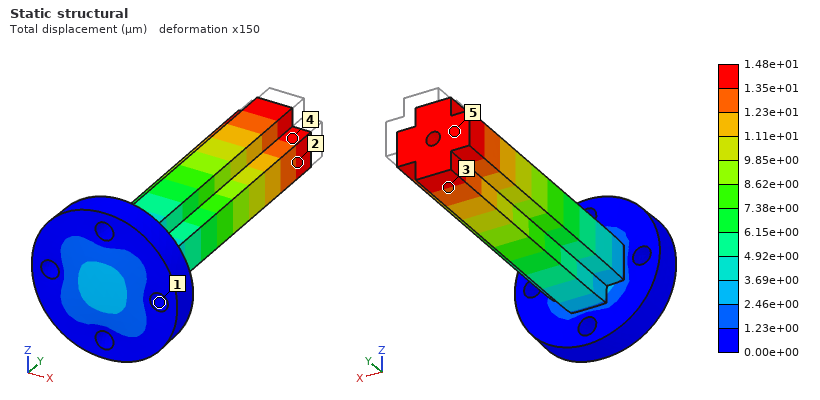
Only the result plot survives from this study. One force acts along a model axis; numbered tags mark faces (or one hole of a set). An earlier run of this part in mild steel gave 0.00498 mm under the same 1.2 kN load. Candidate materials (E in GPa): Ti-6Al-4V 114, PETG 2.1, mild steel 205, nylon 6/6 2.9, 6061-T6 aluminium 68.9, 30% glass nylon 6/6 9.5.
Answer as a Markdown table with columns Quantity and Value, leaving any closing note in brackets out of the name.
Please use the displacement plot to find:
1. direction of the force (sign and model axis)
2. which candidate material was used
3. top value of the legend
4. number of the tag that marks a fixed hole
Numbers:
| Quantity | Value |
|---|---|
| direction of the force | -Y |
| which candidate material was used | 6061-T6 aluminium |
| top value of the legend | 1.48e+01 µm |
| number of the tag that marks a fixed hole | 1 |
